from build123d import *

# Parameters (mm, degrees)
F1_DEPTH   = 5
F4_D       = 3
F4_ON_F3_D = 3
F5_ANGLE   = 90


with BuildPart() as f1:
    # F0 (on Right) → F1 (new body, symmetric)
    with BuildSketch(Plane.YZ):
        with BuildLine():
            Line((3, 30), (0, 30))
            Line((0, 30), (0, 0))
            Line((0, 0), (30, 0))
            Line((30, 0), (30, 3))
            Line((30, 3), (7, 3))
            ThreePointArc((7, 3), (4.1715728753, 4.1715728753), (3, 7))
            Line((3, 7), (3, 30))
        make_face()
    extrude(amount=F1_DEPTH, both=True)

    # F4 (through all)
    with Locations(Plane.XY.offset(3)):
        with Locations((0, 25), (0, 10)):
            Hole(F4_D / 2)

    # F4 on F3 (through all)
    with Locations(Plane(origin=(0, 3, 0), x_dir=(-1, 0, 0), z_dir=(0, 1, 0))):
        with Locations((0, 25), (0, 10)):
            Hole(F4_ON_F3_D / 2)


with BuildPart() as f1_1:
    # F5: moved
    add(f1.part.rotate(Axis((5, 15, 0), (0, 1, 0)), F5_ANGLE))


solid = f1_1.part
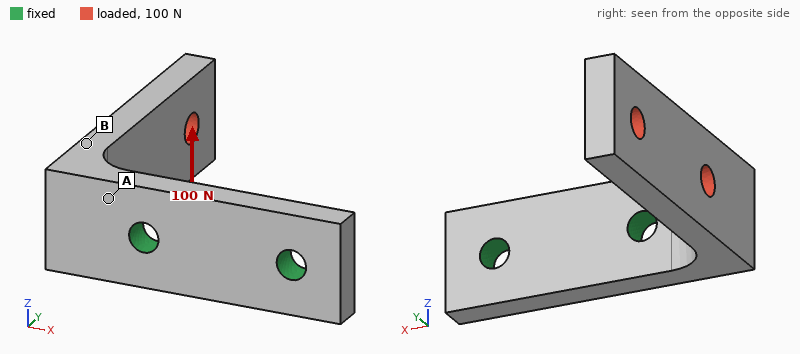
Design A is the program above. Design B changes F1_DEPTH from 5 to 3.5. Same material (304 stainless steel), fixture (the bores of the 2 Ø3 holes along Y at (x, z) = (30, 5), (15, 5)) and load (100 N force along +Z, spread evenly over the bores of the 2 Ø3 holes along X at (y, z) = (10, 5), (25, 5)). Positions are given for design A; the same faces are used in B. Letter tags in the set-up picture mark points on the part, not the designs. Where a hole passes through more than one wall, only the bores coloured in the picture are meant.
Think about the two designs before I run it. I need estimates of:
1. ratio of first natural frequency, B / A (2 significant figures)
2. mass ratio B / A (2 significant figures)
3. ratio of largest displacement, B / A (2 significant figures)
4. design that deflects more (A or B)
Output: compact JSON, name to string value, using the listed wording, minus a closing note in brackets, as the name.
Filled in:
{"ratio of first natural frequency, B / A": "1.0", "mass ratio B / A": "0.68", "ratio of largest displacement, B / A": "1.7", "design that deflects more": "B"}
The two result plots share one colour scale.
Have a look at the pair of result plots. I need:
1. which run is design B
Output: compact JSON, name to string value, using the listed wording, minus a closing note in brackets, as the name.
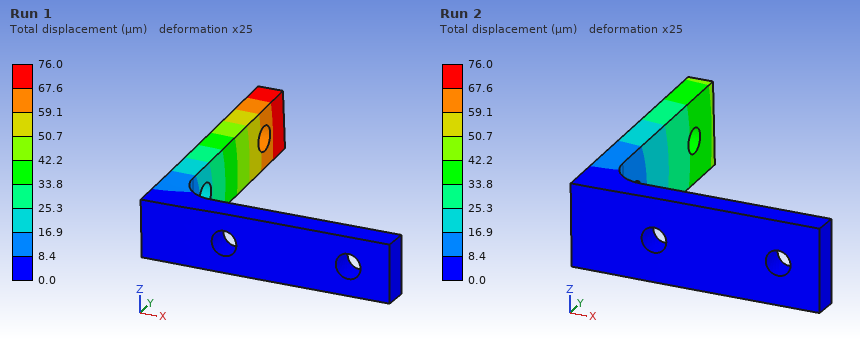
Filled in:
{"which run is design B": "Run 1"}
